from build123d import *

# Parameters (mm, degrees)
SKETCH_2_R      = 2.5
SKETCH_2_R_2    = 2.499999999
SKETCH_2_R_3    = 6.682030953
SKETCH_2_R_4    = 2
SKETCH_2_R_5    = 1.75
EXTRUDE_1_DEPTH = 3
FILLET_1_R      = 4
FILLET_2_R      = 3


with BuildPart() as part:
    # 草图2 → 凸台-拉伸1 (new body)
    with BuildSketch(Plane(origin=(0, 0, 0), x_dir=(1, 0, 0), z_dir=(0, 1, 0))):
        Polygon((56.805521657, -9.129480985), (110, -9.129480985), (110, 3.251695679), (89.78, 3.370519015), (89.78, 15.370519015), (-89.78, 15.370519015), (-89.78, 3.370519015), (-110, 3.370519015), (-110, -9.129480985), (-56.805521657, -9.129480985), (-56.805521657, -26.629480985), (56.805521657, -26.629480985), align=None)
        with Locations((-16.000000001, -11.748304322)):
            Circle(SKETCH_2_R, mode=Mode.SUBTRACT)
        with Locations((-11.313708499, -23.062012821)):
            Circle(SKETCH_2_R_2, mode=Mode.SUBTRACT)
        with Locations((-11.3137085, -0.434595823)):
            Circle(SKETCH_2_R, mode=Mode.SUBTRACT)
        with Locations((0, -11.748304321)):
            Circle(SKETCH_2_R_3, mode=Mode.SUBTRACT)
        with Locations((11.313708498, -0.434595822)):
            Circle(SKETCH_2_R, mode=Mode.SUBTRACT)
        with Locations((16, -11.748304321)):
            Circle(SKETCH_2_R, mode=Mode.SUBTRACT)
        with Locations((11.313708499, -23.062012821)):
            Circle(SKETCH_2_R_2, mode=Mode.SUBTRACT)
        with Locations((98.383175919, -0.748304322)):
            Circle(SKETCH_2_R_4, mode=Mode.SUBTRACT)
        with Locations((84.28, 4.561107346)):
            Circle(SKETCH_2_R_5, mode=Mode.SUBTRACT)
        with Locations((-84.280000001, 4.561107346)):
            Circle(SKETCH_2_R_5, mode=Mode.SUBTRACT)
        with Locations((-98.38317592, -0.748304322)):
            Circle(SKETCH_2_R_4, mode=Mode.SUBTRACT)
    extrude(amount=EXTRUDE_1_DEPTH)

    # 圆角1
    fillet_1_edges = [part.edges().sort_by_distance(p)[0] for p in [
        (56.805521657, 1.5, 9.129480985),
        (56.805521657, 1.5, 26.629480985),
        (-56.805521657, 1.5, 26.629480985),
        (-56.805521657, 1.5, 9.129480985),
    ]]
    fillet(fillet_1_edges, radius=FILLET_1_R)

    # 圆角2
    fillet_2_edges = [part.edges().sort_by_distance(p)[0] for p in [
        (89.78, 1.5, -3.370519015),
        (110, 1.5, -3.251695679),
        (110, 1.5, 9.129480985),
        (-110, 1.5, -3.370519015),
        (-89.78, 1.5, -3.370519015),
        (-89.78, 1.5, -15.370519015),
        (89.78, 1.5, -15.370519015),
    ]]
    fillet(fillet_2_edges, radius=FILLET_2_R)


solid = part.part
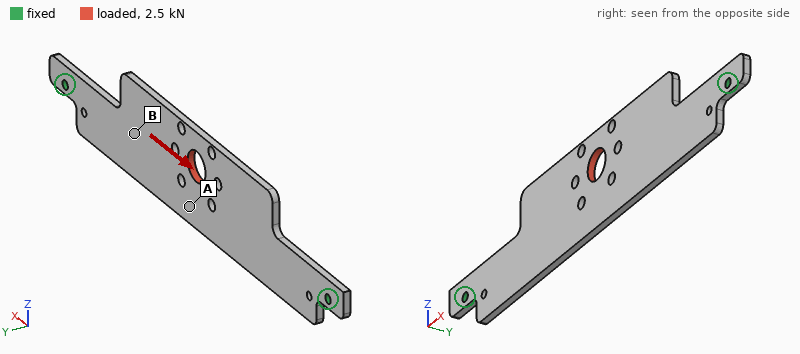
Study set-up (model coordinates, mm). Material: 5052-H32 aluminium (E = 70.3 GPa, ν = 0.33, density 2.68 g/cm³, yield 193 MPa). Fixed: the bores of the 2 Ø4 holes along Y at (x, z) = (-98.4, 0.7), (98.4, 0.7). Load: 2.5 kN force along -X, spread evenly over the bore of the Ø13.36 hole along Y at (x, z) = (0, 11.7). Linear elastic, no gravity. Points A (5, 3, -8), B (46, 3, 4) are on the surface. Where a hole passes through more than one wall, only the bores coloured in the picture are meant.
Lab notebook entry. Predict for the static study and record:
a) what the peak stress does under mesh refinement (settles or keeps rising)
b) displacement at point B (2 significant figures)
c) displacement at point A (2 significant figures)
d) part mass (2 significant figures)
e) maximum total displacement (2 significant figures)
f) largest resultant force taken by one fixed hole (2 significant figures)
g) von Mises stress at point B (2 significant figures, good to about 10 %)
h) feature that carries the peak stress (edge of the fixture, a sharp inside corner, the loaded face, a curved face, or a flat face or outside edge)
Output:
keeps rising
28 µm
22 µm
53 g
39 µm
1.3 kN
20 MPa
edge of the fixture
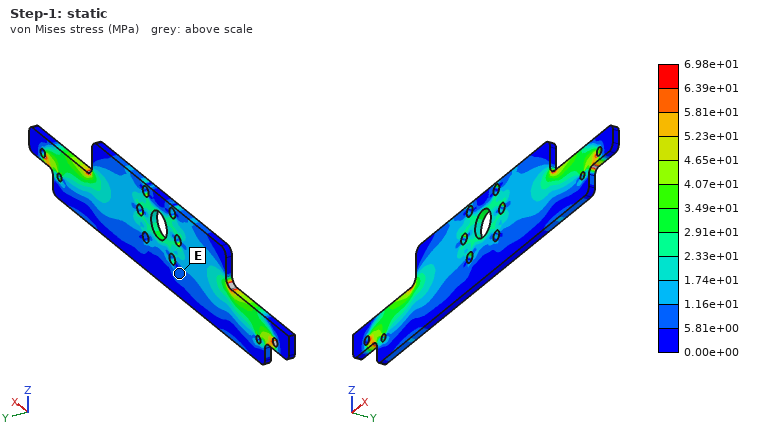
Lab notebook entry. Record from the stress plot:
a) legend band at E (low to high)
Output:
5.81e+00 to 1.16e+01 MPa
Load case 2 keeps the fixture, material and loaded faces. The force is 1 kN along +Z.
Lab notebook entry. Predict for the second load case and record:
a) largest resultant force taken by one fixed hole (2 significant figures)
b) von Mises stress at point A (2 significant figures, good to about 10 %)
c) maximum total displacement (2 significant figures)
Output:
510 N
33 MPa
0.17 mm
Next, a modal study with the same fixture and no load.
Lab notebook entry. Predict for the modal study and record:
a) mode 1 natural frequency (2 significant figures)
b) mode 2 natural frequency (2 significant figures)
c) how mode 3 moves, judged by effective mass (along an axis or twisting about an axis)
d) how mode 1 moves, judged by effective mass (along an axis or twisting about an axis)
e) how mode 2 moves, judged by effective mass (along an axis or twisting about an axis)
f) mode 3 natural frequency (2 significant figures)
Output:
310 Hz
820 Hz
twisting about Z
along Y
twisting about X
940 Hz
